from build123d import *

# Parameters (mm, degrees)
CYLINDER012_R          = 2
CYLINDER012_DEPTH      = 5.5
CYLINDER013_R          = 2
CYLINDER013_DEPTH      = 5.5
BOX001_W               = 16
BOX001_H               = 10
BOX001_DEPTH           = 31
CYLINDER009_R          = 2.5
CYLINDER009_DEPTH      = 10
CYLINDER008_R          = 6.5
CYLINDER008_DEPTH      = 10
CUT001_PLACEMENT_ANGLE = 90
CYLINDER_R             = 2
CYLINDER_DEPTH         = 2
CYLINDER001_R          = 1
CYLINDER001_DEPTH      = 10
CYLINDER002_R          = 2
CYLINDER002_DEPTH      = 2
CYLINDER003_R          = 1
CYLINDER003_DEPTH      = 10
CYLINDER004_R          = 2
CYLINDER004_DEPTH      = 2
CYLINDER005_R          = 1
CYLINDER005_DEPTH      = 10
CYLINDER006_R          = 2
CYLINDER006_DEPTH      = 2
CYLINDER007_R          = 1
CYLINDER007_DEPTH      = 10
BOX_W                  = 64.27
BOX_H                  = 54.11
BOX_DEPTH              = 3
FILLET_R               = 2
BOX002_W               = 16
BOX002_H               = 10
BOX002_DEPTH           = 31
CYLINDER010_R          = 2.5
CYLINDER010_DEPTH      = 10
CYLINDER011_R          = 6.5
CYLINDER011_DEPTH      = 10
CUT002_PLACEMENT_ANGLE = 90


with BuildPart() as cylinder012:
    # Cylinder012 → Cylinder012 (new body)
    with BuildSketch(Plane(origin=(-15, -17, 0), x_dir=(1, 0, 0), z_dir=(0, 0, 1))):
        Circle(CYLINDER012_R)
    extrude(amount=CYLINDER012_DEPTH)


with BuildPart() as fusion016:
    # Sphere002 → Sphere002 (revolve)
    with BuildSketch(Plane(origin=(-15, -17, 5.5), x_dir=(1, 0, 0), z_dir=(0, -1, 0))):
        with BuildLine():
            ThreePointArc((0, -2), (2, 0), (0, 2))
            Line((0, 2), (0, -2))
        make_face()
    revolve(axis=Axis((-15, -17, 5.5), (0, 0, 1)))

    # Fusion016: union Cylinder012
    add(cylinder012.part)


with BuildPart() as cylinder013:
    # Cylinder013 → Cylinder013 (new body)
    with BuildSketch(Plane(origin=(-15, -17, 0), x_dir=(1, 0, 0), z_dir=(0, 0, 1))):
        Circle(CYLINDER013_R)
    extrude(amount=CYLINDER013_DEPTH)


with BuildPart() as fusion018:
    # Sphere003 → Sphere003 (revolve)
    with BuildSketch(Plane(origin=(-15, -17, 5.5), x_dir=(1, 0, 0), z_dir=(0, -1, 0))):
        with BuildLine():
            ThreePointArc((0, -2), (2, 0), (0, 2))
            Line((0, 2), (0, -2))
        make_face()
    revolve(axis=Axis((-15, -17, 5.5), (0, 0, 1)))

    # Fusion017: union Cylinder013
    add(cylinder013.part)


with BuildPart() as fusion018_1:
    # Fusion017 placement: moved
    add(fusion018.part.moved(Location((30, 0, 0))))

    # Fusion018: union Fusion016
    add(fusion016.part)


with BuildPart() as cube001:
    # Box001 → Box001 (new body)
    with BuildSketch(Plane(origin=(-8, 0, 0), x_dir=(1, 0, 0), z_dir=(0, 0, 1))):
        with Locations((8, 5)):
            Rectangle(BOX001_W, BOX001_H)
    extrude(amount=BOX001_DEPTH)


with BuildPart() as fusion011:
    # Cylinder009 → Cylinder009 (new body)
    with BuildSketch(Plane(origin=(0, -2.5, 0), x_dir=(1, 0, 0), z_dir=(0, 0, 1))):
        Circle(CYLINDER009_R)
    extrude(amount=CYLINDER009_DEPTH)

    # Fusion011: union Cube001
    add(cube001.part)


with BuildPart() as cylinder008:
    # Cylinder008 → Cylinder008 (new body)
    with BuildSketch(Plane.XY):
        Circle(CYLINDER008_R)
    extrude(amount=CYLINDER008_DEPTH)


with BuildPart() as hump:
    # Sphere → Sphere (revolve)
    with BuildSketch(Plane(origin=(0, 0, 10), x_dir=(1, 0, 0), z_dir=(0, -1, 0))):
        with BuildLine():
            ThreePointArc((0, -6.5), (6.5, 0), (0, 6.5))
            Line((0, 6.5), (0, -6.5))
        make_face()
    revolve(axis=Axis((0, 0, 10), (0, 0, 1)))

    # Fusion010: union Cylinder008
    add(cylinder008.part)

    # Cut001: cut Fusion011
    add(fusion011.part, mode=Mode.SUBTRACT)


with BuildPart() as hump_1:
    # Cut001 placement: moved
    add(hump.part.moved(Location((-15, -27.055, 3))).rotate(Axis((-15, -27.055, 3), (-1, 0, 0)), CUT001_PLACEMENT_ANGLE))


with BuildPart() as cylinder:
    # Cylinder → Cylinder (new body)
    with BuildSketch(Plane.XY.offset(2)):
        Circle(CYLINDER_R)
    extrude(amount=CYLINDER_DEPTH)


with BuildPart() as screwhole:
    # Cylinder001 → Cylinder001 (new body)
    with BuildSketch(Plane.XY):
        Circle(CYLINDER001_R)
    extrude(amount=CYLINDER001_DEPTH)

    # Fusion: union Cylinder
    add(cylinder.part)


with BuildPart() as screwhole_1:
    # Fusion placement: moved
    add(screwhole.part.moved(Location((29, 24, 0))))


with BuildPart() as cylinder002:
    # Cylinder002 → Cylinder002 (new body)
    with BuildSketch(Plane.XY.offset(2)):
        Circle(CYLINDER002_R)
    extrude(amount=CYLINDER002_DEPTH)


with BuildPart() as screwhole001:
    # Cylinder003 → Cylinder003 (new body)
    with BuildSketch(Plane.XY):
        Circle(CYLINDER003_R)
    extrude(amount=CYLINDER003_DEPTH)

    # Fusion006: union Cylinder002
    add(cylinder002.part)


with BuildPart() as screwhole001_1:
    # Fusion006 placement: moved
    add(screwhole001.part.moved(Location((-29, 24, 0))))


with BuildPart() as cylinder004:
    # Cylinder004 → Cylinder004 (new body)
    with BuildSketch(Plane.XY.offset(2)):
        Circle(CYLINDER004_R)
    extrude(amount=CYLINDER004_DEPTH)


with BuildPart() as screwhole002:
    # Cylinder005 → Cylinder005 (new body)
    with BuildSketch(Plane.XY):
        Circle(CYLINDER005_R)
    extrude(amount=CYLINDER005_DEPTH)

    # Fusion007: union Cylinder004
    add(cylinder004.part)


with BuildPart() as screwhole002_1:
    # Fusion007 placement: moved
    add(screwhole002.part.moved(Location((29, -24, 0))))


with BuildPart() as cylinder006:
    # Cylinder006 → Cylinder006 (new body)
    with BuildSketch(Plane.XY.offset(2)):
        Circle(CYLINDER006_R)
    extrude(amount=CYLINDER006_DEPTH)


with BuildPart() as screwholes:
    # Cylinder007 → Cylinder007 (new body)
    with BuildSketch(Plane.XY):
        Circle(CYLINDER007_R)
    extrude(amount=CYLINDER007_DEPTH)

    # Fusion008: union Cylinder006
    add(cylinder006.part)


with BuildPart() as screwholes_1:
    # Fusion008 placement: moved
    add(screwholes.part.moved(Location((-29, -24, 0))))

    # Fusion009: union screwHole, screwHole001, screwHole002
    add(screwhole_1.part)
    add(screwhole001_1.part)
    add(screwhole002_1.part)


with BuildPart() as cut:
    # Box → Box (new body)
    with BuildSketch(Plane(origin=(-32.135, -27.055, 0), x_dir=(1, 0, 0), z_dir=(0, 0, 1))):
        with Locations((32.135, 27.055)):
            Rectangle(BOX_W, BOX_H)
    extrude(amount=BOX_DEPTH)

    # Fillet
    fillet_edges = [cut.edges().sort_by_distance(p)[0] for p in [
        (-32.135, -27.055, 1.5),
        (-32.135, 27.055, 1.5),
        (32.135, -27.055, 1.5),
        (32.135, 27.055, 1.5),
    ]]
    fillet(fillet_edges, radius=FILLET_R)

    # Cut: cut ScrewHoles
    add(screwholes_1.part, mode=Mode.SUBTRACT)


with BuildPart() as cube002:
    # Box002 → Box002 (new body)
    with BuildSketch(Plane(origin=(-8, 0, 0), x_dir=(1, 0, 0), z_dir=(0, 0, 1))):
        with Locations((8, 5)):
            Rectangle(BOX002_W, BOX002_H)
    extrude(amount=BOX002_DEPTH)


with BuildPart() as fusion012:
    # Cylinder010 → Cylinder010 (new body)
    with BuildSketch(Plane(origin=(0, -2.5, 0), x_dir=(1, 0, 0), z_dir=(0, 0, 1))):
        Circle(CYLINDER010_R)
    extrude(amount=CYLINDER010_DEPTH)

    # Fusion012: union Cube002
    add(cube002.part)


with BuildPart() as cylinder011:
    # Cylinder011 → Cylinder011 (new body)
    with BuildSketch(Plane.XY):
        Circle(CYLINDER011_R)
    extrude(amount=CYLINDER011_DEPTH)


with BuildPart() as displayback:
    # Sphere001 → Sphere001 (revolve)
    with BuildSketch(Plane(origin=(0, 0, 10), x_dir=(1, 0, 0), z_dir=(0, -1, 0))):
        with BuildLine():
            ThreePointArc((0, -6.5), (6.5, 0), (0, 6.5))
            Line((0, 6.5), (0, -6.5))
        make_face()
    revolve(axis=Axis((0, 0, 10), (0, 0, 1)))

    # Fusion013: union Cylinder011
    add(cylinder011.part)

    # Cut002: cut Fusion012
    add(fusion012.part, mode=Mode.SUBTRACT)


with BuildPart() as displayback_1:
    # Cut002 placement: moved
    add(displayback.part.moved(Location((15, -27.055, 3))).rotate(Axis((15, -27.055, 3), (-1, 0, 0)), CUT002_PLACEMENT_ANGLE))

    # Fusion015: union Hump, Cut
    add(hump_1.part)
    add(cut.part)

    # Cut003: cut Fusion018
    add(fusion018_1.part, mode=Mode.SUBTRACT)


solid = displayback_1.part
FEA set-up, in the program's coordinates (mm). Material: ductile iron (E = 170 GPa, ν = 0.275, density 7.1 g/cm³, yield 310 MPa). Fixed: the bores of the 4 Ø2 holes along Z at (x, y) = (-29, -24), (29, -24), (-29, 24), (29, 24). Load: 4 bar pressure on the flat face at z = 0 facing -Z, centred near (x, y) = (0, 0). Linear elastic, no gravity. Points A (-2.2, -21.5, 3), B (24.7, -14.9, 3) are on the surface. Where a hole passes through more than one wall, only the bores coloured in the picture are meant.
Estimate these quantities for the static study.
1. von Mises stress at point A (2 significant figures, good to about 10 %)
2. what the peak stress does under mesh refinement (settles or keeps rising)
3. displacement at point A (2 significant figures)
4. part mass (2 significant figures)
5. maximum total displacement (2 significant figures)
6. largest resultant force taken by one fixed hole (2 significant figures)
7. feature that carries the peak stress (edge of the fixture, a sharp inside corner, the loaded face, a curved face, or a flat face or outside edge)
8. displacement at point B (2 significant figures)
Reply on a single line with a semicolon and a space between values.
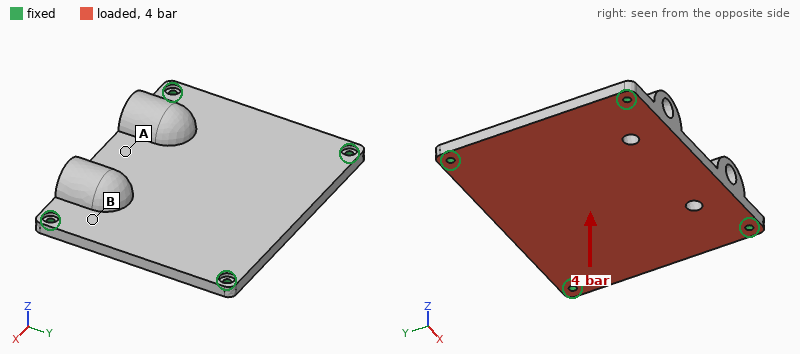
68 MPa; keeps rising; 63 µm; 83 g; 88 µm; 490 N; edge of the fixture; 27 µm
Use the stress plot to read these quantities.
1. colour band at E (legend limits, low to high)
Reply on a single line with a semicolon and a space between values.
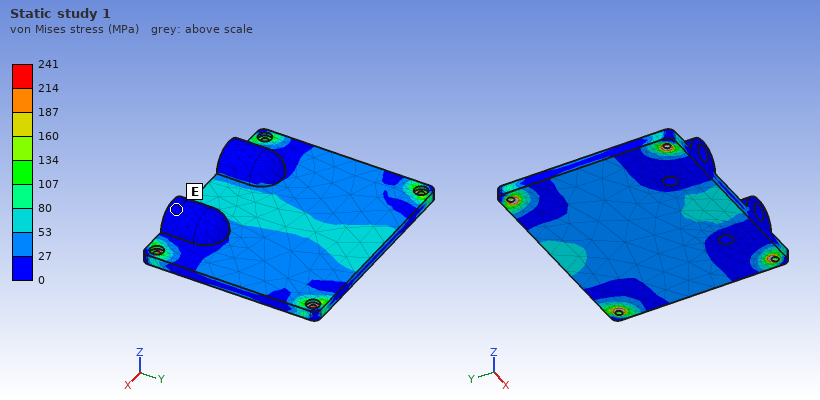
0 to 27 MPa
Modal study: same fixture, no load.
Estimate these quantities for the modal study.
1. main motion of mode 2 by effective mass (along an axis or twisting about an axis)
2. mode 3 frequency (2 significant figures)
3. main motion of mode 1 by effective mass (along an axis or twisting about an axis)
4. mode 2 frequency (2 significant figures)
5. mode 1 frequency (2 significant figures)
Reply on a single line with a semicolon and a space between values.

twisting about X; 5700 Hz; along Z; 4600 Hz; 2600 Hz
